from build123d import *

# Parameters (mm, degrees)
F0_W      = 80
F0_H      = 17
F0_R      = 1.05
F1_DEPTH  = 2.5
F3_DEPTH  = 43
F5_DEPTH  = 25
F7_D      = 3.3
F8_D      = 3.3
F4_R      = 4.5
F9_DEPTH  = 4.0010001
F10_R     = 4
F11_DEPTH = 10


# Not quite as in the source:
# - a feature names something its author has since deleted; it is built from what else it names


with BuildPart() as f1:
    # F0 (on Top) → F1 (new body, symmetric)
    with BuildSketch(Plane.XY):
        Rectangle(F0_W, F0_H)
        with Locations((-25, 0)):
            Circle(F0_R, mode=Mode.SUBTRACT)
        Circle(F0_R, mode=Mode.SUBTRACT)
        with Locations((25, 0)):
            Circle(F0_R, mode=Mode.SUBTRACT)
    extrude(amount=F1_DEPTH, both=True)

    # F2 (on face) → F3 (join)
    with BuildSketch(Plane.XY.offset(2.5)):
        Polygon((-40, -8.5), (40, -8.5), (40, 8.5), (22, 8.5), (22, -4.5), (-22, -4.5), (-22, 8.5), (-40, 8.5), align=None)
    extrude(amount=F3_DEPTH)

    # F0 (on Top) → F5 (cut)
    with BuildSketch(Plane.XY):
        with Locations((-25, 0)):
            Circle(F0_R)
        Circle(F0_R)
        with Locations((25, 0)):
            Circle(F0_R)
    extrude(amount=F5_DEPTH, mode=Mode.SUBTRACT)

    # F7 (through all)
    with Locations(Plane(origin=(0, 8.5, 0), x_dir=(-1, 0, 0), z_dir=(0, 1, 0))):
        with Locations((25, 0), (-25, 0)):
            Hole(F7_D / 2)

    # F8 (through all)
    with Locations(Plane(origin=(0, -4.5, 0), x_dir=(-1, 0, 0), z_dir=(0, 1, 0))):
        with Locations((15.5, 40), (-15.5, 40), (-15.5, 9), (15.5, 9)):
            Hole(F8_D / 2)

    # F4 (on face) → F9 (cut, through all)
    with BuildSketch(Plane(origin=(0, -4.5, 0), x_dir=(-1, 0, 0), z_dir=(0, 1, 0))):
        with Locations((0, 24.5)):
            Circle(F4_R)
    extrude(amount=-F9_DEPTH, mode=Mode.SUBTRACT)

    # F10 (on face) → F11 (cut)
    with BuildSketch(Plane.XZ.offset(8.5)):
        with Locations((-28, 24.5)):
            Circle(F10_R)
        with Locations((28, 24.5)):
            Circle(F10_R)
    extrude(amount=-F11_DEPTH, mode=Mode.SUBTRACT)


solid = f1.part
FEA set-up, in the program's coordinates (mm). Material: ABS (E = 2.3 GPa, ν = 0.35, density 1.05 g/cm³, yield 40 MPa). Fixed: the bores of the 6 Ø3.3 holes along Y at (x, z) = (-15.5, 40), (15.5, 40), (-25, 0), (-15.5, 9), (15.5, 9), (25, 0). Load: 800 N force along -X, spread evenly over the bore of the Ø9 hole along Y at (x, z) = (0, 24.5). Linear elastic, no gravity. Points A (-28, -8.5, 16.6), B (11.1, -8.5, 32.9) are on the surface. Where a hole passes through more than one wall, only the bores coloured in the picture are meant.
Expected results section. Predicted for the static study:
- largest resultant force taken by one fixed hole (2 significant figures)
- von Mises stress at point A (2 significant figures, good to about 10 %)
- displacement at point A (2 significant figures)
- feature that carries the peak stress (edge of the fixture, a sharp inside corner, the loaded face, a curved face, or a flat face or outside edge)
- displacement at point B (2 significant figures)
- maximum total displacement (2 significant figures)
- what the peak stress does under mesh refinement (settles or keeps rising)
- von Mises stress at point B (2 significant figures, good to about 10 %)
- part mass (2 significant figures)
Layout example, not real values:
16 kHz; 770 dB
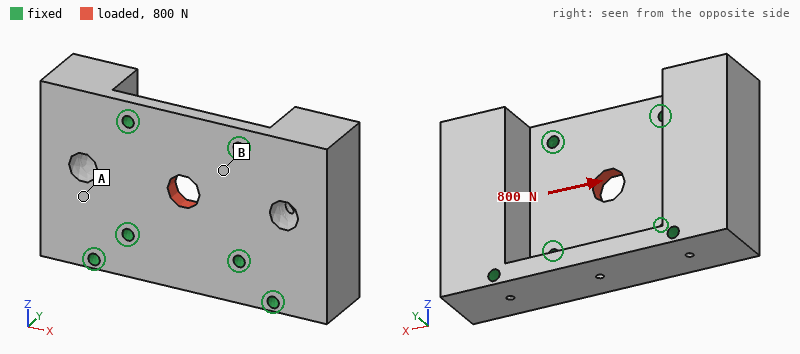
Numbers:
210 N; 1.1 MPa; 12 µm; edge of the fixture; 19 µm; 46 µm; keeps rising; 3.9 MPa; 41 g
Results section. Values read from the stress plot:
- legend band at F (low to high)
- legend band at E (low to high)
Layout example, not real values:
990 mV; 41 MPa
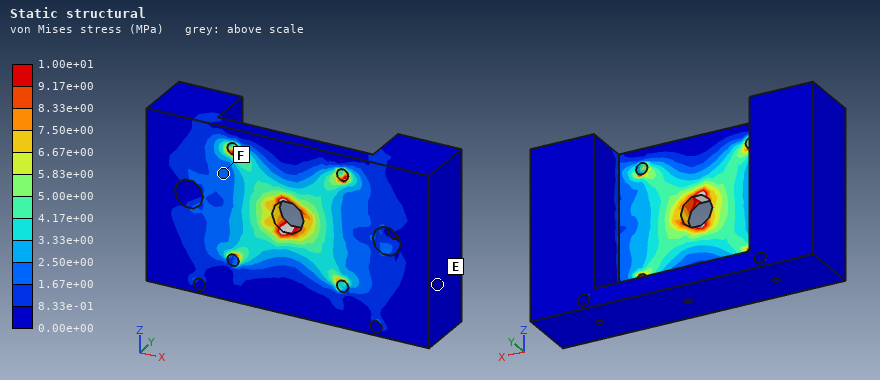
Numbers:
1.67e+00 to 2.50e+00 MPa; 0.00e+00 to 8.33e-01 MPa
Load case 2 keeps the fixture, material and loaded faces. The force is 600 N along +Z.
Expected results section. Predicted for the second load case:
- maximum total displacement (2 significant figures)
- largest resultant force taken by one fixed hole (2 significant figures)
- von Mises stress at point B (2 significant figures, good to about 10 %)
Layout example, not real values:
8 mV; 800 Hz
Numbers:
42 µm; 150 N; 3.5 MPa
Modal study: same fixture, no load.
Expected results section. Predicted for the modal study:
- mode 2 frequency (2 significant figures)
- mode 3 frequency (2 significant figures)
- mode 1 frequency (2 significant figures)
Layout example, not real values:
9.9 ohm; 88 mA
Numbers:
2300 Hz; 4500 Hz; 2300 Hz
